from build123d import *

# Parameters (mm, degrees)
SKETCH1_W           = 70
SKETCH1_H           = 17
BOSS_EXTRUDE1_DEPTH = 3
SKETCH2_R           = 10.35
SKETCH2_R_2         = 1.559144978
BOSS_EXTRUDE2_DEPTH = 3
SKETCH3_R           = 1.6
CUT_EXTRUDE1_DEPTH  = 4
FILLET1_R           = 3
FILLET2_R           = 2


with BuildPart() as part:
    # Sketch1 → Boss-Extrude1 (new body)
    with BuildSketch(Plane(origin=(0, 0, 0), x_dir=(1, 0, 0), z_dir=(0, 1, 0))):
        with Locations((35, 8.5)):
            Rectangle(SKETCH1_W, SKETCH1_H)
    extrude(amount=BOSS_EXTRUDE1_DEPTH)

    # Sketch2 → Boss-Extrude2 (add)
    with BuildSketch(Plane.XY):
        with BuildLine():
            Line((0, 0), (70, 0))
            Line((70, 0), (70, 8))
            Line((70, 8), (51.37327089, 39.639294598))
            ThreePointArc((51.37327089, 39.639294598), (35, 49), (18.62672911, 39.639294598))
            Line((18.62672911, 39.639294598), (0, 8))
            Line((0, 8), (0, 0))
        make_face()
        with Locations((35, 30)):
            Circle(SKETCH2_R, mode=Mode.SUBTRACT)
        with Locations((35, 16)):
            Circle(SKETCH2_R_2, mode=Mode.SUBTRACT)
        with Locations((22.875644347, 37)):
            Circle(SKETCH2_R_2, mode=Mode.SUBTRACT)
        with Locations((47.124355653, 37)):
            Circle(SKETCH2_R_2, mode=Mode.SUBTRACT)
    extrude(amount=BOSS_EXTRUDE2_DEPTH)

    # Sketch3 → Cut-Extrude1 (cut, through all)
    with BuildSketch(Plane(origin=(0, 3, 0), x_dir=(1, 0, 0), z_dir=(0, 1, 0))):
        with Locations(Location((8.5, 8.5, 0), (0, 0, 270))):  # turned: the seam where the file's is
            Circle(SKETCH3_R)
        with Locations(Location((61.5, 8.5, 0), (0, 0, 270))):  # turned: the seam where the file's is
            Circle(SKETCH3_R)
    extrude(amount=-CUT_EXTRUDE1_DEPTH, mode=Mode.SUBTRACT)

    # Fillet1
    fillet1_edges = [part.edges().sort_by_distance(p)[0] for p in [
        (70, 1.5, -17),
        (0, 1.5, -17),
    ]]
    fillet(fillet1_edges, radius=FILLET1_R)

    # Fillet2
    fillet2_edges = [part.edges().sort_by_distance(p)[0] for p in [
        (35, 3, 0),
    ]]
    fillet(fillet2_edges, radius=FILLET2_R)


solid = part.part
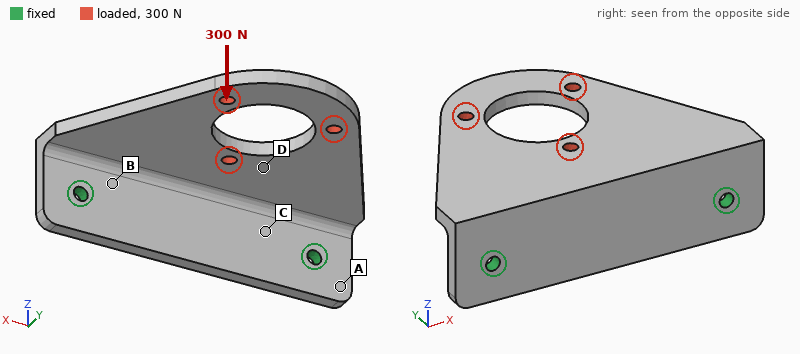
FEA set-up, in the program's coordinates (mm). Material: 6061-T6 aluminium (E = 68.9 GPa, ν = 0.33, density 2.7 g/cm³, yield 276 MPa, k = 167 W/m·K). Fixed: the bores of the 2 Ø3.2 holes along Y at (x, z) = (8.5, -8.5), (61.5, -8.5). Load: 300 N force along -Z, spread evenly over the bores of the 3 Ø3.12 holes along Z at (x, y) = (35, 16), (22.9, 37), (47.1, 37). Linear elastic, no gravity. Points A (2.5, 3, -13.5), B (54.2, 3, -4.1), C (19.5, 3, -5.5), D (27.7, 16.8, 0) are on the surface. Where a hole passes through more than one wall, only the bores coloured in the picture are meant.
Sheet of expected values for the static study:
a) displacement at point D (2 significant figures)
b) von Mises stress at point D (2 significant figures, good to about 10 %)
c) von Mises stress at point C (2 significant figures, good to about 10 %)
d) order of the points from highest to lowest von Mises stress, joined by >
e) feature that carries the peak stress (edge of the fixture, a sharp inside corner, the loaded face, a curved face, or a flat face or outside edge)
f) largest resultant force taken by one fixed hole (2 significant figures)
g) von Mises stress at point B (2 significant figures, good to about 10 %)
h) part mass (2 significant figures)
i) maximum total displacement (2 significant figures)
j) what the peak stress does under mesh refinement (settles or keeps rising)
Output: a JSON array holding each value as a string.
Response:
["0.24 mm", "44 MPa", "65 MPa", "B > C > D > A", "edge of the fixture", "170 N", "82 MPa", "26 g", "1.1 mm", "keeps rising"]
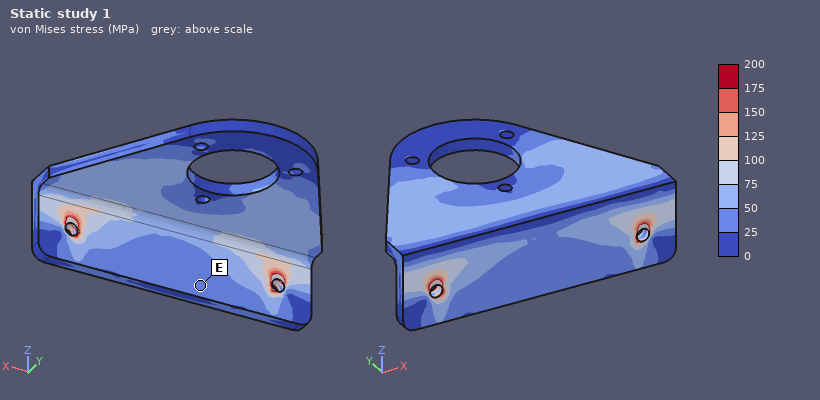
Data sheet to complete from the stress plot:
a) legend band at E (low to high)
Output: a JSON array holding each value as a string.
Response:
["25 to 50 MPa"]
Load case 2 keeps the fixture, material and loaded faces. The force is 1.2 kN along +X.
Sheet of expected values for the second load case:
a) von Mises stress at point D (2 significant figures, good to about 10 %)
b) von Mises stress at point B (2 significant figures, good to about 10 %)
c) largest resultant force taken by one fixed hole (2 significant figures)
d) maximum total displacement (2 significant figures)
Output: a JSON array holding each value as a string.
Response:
["32 MPa", "58 MPa", "900 N", "0.14 mm"]
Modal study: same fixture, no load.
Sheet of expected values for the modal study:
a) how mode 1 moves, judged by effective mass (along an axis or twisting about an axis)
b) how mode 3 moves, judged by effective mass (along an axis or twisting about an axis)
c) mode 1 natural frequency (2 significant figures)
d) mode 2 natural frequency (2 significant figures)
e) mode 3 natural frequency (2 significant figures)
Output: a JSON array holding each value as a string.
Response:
["along Z", "along Y", "1200 Hz", "3300 Hz", "4500 Hz"]
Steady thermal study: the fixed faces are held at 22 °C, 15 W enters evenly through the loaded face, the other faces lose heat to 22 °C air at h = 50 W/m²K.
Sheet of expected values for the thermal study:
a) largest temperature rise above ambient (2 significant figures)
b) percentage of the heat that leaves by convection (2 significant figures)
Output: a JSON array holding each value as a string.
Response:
["28 K", "25 %"]
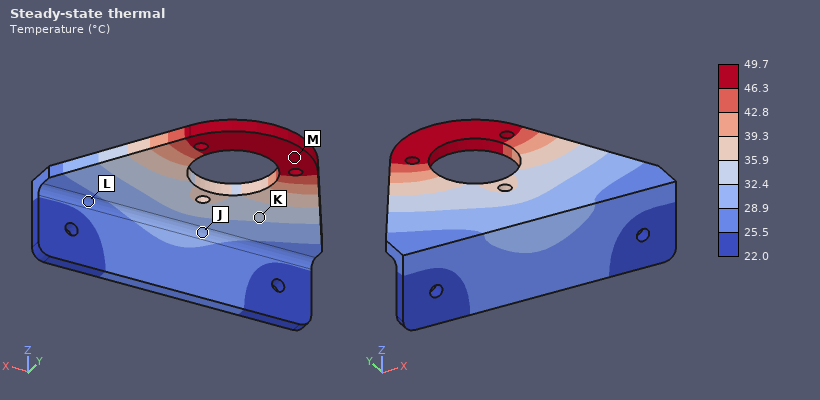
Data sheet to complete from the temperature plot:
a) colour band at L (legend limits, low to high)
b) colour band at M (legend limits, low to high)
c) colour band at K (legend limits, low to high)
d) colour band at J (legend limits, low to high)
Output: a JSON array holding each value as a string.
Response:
["25.5 to 28.9 °C", "46.3 to 49.7 °C", "32.4 to 35.9 °C", "28.9 to 32.4 °C"]
